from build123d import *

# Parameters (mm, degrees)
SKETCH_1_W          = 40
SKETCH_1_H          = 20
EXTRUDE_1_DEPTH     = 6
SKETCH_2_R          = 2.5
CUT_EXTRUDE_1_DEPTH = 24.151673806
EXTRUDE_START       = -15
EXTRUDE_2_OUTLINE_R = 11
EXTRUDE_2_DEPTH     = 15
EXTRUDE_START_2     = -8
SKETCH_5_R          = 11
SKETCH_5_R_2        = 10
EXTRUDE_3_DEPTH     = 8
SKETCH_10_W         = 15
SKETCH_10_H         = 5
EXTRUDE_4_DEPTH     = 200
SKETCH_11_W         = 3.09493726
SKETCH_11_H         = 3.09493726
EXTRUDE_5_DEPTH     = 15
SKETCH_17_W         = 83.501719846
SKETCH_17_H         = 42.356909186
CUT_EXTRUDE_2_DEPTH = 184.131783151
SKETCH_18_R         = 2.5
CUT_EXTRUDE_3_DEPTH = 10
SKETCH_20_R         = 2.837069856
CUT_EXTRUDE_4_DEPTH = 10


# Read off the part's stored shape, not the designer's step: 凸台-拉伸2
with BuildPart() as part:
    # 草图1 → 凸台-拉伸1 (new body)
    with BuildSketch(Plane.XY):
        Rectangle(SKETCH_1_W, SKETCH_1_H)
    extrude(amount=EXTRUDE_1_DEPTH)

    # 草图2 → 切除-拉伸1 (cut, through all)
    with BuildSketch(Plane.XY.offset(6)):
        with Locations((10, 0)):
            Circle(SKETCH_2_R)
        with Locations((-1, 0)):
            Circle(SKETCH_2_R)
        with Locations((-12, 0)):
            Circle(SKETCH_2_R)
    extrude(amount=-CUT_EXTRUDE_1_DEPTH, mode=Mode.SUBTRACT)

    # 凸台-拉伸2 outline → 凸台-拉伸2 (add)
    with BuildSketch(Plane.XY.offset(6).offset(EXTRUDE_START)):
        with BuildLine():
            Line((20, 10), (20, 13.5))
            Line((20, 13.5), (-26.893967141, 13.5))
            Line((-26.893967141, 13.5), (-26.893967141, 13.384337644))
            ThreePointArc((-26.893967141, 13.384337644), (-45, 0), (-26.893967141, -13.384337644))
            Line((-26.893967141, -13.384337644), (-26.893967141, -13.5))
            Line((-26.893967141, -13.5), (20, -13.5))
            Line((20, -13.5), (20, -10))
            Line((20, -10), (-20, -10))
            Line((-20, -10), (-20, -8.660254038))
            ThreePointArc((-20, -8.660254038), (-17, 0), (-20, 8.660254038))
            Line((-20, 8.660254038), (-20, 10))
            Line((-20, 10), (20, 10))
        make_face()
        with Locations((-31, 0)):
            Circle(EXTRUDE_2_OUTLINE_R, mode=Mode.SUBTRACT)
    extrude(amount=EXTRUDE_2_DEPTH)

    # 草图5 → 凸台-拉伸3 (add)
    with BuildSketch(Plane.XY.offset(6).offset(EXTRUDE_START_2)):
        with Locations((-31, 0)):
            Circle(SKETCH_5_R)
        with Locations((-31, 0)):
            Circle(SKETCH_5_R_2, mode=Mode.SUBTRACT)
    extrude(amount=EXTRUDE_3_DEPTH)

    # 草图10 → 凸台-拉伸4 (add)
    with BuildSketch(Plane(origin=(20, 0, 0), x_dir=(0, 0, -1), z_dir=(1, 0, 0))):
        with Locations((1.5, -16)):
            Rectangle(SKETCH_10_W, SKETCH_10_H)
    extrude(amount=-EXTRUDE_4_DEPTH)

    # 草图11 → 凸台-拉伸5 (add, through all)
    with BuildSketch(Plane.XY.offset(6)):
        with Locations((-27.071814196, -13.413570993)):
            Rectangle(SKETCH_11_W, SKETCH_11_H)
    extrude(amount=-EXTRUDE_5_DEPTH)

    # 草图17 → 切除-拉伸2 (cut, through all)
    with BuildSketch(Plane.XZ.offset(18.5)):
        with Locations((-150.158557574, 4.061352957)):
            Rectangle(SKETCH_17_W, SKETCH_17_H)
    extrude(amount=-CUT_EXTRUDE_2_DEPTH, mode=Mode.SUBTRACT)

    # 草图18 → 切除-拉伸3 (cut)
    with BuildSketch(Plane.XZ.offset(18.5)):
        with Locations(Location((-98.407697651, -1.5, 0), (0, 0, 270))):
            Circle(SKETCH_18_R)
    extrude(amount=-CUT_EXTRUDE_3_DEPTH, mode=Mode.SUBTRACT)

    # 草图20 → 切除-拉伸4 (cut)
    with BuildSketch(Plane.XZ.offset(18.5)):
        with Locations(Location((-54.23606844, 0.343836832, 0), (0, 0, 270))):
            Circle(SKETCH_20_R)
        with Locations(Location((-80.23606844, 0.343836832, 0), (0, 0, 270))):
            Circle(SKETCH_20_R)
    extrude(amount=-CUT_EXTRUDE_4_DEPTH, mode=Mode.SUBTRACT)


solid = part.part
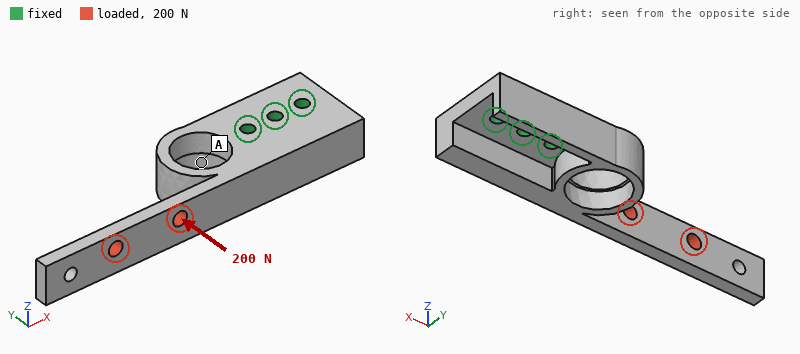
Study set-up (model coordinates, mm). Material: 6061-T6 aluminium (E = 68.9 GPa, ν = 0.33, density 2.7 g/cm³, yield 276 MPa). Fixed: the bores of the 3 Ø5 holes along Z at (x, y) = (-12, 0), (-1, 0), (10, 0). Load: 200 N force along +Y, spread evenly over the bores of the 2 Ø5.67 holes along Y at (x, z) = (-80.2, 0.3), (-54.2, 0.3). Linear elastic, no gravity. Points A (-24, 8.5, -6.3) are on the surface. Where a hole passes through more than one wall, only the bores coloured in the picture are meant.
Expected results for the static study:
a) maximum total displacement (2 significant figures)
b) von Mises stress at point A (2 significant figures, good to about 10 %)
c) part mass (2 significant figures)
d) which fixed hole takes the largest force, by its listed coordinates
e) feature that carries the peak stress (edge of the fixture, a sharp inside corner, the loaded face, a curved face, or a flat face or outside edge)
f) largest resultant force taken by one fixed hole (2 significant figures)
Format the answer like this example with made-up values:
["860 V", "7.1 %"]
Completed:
["0.98 mm", "10 MPa", "60 g", "(-12, 0)", "the loaded face", "690 N"]
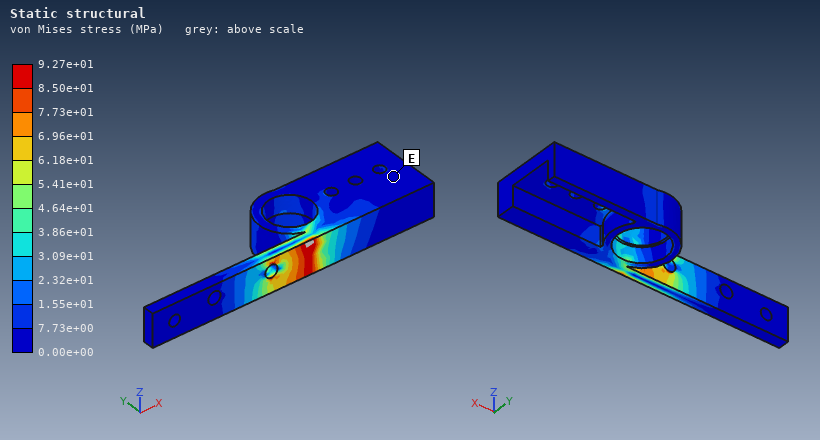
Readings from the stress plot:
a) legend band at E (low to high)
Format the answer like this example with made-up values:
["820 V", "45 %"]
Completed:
["0.00e+00 to 7.73e+00 MPa"]
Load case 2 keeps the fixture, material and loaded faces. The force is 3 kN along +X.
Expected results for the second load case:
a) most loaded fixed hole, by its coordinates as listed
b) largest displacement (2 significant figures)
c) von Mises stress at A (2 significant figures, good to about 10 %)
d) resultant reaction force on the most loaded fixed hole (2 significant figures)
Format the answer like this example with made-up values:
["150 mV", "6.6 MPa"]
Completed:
["(-12, 0)", "0.24 mm", "9.9 MPa", "2.2 kN"]
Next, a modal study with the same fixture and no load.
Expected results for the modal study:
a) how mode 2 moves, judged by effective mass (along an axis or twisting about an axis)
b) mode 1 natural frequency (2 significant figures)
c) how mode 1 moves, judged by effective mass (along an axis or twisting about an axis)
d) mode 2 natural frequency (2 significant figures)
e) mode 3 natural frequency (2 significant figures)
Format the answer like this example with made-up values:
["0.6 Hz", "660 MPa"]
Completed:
["along Z", "660 Hz", "along Y", "1400 Hz", "3800 Hz"]
